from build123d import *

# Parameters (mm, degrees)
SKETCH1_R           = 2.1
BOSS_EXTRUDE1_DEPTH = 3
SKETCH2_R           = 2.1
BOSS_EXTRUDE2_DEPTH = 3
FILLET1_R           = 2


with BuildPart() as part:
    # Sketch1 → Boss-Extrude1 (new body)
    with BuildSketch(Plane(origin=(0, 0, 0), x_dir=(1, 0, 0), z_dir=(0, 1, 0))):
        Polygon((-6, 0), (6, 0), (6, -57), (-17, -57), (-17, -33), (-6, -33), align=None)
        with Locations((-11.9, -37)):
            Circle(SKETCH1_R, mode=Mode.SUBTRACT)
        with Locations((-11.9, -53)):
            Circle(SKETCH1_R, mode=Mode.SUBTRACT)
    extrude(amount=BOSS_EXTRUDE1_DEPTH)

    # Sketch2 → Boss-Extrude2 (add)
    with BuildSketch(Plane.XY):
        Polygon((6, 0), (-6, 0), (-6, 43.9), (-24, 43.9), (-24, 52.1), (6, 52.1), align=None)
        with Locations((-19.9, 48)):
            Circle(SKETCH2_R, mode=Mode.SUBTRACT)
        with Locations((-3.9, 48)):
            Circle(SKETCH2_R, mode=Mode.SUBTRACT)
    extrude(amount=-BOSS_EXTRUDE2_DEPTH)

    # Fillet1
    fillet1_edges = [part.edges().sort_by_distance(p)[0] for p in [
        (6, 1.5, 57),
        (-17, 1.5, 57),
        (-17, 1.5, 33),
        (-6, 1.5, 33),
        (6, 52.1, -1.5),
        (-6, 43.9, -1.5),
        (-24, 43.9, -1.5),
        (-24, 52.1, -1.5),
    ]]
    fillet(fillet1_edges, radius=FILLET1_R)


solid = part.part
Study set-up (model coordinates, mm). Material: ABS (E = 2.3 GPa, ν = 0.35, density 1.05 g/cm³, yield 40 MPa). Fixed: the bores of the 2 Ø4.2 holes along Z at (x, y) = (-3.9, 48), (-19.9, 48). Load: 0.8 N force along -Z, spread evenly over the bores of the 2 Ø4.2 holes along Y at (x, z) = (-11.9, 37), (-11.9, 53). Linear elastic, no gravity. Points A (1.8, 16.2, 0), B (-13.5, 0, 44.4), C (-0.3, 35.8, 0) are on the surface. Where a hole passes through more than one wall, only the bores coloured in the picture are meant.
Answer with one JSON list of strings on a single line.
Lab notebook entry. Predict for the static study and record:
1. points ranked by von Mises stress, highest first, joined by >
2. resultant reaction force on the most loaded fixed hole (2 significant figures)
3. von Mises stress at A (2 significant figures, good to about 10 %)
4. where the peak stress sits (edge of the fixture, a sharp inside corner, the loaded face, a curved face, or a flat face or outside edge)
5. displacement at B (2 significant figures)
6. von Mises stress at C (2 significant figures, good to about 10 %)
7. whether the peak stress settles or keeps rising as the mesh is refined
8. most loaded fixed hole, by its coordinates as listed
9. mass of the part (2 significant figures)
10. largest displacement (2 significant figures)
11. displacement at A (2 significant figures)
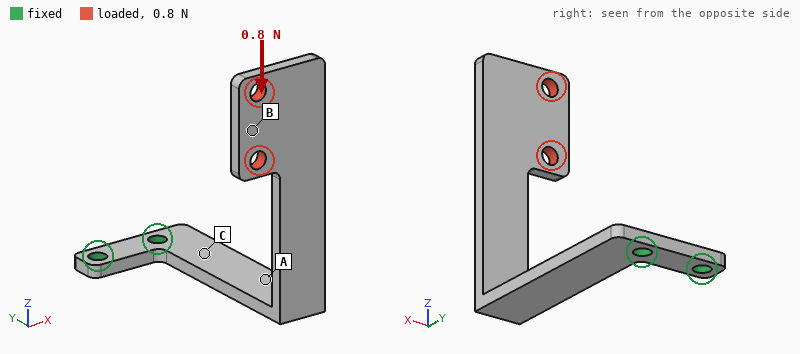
["C > A > B", "1.0 N", "0.82 MPa", "edge of the fixture", "0.82 mm", "1.6 MPa", "keeps rising", "(-3.9, 48)", "5.2 g", "0.97 mm", "0.21 mm"]
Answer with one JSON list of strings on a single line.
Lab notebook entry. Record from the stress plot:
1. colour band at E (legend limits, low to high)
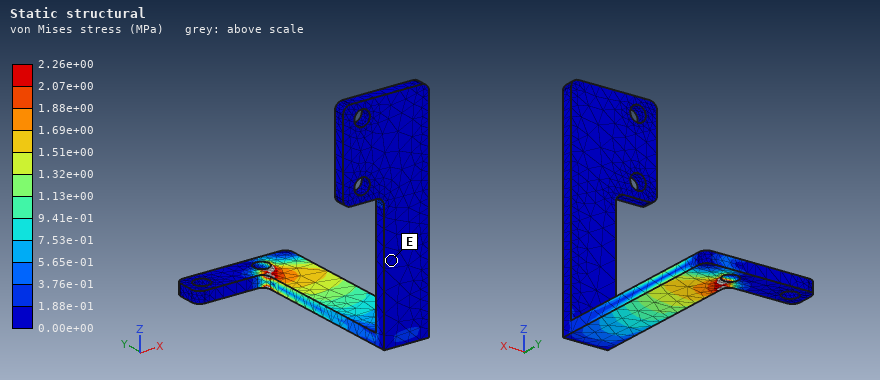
["0.00e+00 to 1.88e-01 MPa"]
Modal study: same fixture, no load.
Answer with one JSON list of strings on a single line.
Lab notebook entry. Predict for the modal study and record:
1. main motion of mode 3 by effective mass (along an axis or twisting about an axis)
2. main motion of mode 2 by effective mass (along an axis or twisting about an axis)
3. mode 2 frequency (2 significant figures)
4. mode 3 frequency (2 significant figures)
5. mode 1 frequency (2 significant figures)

["along Z", "along X", "99 Hz", "210 Hz", "71 Hz"]
